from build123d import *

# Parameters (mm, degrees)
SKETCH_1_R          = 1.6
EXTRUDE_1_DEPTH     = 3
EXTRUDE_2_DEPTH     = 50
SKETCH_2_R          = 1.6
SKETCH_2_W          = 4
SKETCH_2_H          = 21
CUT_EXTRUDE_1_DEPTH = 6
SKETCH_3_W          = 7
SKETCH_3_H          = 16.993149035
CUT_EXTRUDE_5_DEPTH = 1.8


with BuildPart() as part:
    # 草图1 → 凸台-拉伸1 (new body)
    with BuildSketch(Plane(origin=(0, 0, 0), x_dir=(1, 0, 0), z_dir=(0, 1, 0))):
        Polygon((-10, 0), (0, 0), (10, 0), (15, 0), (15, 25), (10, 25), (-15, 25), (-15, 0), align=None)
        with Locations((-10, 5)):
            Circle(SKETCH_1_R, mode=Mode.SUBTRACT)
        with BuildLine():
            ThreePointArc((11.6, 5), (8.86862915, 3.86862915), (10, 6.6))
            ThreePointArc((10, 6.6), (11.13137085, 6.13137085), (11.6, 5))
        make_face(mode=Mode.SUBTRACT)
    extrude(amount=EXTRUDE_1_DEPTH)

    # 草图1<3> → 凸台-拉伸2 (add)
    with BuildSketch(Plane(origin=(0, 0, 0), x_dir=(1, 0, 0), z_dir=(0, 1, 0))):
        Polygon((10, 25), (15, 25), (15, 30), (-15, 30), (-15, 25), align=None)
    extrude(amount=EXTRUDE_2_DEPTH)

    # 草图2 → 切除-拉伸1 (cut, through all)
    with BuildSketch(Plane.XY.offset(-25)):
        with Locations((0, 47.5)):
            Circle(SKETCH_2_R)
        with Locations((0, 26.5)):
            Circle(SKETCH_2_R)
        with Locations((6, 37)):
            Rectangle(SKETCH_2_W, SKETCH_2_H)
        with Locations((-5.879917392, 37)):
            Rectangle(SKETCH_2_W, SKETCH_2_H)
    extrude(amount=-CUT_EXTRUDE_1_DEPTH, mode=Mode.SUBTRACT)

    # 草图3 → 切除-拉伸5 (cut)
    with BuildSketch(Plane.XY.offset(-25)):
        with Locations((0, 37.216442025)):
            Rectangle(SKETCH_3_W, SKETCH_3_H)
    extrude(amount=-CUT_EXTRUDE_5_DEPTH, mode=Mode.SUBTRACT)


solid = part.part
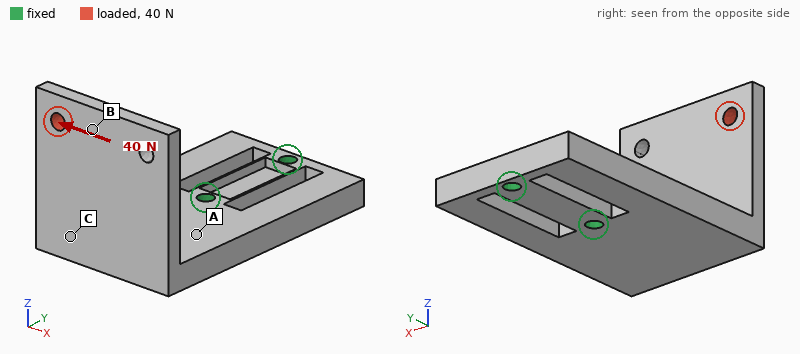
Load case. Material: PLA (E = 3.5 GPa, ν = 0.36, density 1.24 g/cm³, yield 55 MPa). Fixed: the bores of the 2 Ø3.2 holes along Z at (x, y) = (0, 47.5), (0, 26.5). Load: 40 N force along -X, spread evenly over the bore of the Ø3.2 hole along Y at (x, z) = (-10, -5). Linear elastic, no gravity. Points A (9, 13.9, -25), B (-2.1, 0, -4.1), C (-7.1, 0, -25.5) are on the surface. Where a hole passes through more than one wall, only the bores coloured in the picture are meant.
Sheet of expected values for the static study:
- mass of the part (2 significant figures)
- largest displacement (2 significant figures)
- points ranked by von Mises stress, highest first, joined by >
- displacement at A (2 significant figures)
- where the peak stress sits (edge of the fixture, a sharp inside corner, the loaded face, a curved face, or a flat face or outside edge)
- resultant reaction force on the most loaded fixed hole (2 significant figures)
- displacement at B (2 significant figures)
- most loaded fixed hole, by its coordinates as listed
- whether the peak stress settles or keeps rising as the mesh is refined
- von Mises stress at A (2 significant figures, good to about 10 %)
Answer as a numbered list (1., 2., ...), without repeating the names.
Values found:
1. 11 g
2. 0.67 mm
3. A > C > B
4. 0.13 mm
5. edge of the fixture
6. 67 N
7. 0.52 mm
8. (0, 26.5)
9. keeps rising
10. 6.0 MPa
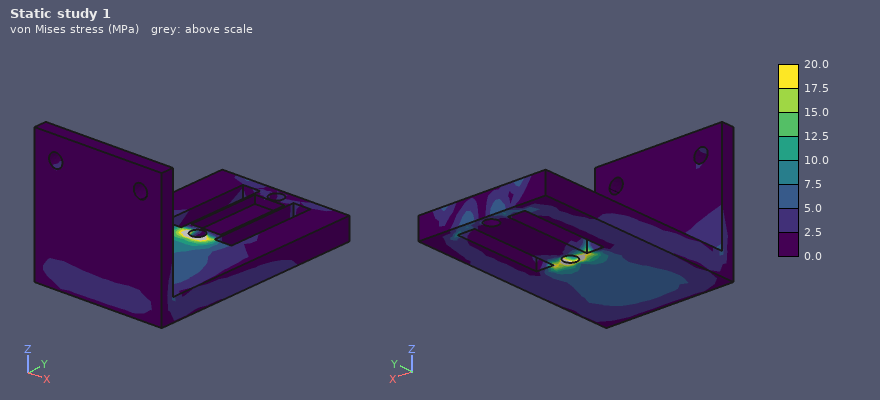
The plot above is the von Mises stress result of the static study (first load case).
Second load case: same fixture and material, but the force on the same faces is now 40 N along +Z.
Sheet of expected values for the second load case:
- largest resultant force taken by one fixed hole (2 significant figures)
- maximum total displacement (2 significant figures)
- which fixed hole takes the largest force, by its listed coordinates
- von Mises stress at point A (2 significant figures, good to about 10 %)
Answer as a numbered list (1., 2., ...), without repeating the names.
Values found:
1. 55 N
2. 0.63 mm
3. (0, 26.5)
4. 4.3 MPa
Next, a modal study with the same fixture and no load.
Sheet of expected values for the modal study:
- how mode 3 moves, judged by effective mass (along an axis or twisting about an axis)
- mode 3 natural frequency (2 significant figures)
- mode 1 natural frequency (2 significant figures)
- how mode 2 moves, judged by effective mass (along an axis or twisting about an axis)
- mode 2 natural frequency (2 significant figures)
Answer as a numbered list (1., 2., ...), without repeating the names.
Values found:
1. along Z
2. 1500 Hz
3. 710 Hz
4. along X
5. 960 Hz
